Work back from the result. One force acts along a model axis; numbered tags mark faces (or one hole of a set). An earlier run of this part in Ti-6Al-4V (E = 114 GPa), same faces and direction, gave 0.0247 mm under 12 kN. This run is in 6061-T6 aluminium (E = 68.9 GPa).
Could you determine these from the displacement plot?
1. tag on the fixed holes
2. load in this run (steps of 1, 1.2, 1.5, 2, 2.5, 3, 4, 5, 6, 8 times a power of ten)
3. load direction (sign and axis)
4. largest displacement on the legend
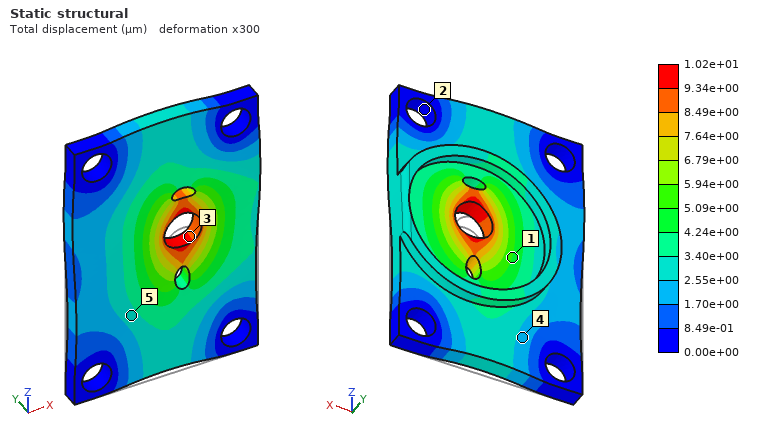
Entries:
2
3 kN
+Z
1.02e+01 µm
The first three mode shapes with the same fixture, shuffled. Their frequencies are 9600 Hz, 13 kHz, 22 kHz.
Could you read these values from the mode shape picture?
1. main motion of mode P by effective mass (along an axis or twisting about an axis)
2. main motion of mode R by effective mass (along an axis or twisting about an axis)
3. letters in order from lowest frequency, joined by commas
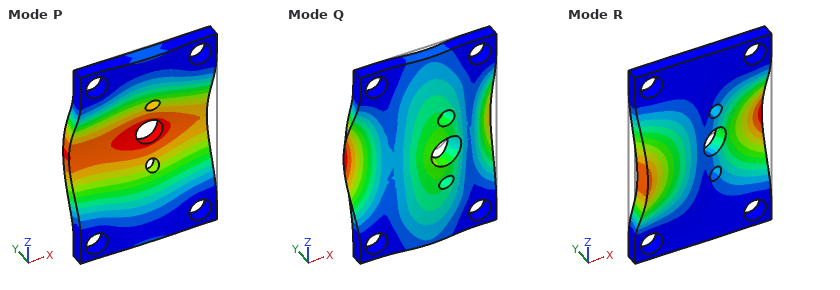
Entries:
along Y
twisting about Z
P, R, Q
